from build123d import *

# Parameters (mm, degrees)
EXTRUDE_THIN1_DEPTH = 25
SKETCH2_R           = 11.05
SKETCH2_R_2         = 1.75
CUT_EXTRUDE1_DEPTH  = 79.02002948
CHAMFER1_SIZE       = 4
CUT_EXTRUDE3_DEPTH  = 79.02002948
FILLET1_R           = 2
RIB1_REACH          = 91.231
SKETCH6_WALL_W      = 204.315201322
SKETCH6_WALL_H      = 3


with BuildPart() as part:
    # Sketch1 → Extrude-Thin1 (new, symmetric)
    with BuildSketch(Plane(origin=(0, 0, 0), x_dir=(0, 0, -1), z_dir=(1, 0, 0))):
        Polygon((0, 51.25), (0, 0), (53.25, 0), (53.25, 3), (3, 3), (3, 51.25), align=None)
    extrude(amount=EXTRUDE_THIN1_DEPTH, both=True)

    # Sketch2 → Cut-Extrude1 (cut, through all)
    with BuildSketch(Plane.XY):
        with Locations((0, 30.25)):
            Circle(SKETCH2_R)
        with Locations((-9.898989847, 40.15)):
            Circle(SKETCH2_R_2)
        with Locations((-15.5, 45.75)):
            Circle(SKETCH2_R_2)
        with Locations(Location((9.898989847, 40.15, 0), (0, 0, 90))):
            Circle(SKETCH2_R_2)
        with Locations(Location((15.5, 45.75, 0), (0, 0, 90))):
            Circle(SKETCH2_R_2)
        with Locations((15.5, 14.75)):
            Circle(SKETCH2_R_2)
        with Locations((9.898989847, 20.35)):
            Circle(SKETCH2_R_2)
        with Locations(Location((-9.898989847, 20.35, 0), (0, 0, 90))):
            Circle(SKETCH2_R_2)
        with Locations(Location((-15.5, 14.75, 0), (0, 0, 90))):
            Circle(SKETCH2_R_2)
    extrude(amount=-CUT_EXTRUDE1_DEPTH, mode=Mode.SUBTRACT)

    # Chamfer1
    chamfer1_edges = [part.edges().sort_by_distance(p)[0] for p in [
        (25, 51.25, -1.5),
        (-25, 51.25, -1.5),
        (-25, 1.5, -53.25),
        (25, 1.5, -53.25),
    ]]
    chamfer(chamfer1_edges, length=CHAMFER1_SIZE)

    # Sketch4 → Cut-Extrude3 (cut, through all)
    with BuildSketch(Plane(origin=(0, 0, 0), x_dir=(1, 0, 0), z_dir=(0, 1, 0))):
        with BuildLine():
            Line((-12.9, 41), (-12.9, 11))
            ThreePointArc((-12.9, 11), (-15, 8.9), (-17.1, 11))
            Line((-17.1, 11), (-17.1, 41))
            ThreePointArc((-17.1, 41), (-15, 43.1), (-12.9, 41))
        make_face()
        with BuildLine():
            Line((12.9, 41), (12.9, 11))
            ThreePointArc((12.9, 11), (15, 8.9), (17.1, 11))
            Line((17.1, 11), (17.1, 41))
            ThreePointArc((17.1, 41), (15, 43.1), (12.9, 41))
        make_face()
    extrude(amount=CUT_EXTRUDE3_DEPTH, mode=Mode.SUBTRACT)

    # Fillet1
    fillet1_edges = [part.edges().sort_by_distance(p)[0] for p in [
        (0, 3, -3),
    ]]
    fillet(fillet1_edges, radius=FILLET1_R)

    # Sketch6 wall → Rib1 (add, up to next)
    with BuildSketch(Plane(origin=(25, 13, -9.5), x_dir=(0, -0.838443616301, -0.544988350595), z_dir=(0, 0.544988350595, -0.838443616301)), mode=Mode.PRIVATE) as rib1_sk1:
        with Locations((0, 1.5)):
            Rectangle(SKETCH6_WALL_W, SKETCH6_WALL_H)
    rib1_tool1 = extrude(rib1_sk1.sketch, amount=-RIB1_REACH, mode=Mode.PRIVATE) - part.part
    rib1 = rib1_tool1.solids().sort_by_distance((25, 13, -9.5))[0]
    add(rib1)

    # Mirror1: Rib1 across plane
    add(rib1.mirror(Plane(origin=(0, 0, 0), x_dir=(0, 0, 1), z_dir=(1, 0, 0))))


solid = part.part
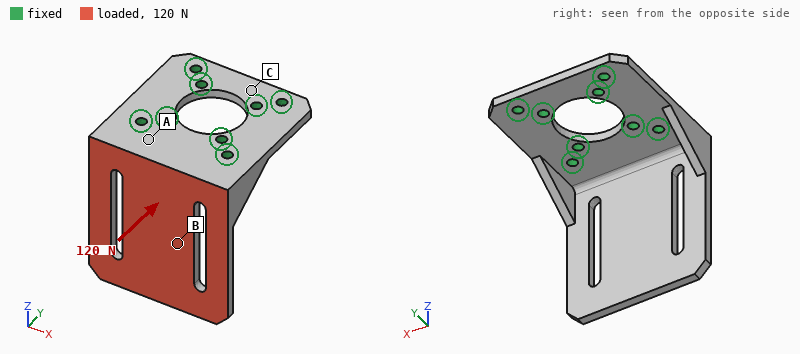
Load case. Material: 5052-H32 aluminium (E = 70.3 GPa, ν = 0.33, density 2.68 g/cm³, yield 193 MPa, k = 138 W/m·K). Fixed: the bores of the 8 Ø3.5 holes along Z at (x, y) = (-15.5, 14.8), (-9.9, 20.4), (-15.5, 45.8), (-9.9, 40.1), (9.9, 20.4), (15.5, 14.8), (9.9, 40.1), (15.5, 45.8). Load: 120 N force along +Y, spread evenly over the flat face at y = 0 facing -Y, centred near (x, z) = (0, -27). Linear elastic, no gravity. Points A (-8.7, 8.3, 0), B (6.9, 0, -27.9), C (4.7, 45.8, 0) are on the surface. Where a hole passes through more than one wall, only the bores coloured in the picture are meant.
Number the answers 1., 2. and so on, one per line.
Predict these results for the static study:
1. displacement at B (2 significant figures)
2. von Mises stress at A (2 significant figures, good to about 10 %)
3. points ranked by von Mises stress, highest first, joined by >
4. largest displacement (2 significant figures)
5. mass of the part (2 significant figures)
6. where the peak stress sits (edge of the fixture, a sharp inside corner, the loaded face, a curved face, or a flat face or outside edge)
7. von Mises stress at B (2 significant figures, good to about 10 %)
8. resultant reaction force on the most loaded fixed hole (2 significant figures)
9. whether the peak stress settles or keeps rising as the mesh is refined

1. 0.11 mm
2. 15 MPa
3. A > B > C
4. 0.27 mm
5. 37 g
6. edge of the fixture
7. 8.5 MPa
8. 81 N
9. keeps rising
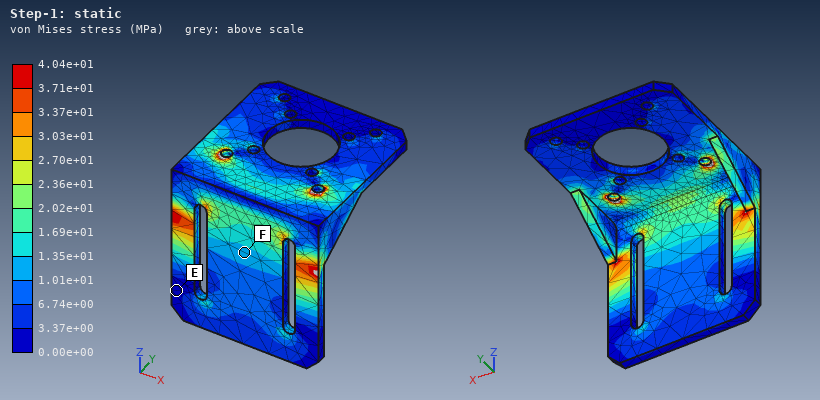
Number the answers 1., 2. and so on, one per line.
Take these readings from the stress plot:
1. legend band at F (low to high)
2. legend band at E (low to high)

1. 1.01e+01 to 1.35e+01 MPa
2. 0.00e+00 to 3.37e+00 MPa
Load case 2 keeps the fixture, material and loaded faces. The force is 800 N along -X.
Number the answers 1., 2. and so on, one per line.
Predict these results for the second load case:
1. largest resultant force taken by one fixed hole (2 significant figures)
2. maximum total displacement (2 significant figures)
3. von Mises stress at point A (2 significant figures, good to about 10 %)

1. 820 N
2. 0.21 mm
3. 33 MPa
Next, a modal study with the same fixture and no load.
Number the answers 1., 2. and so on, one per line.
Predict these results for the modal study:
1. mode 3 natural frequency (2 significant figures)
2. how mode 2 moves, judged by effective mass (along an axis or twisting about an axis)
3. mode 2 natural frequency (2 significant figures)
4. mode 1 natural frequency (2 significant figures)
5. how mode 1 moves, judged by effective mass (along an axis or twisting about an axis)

1. 3200 Hz
2. along X
3. 2200 Hz
4. 950 Hz
5. along Y
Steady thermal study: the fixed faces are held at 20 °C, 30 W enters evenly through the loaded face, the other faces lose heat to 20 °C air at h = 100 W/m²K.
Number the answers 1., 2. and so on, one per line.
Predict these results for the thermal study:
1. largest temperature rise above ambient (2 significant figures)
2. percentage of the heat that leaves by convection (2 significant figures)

1. 36 K
2. 34 %
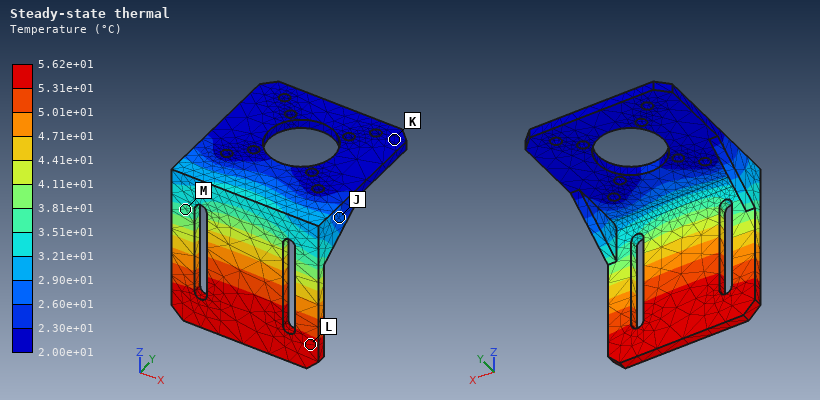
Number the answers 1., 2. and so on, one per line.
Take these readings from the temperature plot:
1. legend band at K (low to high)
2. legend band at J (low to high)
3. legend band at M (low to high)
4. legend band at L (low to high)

1. 2.00e+01 to 2.30e+01 °C
2. 2.60e+01 to 2.90e+01 °C
3. 3.51e+01 to 3.81e+01 °C
4. 5.31e+01 to 5.62e+01 °C
